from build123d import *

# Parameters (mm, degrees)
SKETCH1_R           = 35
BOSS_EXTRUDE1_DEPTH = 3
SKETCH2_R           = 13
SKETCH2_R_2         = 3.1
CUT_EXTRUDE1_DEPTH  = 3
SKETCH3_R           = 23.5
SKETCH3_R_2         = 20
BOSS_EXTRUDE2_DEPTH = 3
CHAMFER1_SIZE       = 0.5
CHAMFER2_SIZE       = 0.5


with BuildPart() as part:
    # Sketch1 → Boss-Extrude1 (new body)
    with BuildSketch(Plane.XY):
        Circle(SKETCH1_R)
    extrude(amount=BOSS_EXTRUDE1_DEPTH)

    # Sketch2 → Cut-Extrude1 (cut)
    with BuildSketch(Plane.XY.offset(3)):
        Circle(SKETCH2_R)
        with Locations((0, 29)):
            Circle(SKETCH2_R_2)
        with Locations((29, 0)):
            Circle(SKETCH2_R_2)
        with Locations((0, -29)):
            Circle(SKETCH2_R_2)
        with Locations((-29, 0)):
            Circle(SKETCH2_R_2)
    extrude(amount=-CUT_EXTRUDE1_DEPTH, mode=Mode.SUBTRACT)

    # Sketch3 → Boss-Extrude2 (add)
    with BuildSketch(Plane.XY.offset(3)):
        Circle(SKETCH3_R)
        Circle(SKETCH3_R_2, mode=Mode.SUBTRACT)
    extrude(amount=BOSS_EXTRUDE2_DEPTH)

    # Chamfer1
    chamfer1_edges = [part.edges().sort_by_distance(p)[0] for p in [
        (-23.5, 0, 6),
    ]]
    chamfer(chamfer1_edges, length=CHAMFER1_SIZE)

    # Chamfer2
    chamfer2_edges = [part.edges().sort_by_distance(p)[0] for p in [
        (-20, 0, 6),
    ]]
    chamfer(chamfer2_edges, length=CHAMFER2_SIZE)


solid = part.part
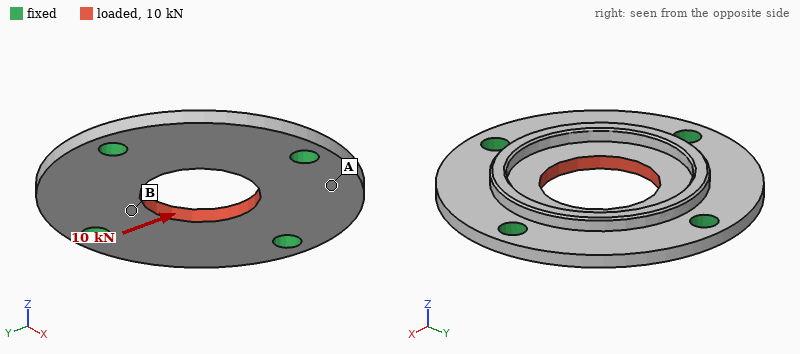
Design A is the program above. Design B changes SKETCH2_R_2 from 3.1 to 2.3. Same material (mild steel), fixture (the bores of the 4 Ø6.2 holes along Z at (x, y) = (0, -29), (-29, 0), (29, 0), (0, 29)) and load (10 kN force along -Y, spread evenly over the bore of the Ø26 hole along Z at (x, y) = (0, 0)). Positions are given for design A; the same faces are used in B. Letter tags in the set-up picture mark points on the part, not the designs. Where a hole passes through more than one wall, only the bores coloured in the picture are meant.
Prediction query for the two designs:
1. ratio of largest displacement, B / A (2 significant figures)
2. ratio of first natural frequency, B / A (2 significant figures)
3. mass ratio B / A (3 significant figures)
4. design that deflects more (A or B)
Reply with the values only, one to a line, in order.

1.1
0.89
1.01
B
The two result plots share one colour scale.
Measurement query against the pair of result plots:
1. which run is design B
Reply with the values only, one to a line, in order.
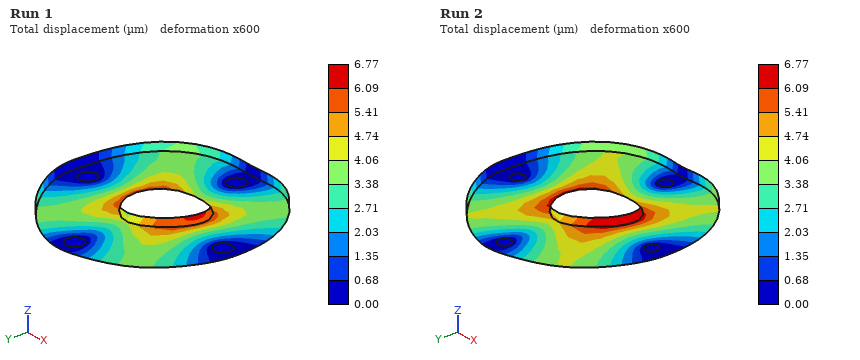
Run 2
